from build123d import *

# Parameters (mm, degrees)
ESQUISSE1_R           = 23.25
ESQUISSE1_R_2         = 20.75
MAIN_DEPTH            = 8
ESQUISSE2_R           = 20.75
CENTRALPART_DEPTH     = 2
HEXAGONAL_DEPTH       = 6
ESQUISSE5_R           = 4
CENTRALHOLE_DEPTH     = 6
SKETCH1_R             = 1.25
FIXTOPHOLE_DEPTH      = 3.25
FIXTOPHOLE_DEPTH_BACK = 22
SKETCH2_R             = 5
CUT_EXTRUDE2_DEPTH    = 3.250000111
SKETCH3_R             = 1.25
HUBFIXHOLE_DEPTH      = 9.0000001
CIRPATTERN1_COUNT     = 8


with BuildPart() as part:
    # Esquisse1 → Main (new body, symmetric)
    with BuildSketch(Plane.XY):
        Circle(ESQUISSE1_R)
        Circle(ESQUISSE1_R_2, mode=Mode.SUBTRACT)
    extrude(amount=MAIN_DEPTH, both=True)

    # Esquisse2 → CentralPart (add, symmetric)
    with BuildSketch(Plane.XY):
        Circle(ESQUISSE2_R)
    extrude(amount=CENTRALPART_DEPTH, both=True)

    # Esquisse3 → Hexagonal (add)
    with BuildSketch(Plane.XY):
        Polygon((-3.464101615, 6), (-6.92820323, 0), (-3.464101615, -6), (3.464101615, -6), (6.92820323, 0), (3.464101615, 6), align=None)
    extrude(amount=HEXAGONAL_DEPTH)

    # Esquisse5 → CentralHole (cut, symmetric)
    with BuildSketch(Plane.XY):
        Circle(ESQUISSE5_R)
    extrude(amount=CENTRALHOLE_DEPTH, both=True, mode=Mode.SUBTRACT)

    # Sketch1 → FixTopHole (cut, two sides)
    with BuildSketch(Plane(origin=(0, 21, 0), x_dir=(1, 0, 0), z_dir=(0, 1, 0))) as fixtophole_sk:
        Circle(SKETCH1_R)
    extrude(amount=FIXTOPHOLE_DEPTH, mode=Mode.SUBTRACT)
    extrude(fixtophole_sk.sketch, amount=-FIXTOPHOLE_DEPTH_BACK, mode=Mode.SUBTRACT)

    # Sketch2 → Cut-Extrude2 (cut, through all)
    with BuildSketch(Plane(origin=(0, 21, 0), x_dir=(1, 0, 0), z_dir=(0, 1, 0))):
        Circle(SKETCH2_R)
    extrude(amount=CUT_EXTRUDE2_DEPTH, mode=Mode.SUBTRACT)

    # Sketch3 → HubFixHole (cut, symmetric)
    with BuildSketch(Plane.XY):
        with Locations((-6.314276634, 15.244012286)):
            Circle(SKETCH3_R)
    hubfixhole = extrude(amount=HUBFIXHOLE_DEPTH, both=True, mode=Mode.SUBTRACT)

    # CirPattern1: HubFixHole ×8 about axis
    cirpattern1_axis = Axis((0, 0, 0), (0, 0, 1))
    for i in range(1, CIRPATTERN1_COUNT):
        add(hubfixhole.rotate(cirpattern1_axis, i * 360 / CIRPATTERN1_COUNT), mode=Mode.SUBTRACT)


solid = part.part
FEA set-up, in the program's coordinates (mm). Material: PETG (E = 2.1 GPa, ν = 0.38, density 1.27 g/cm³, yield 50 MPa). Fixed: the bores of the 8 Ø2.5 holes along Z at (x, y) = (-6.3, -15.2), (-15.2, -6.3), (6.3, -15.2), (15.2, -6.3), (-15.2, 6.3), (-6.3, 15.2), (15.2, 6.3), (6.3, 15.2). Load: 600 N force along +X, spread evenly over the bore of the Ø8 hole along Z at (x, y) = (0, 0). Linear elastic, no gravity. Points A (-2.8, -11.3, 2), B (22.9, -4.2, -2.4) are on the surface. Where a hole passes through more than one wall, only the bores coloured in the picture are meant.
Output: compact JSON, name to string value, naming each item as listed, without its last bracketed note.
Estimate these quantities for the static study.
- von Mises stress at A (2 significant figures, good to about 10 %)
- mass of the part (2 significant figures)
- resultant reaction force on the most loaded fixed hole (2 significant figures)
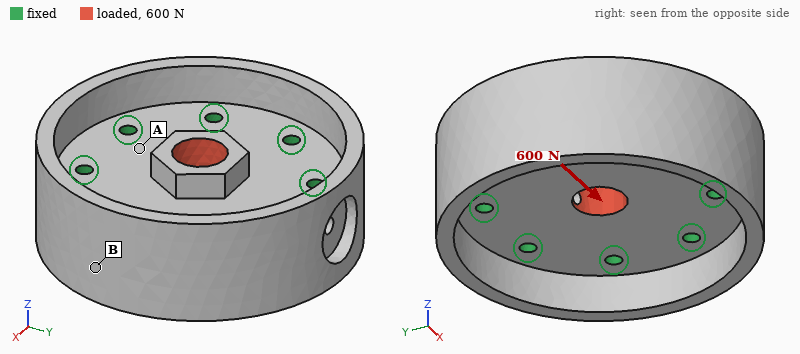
{"von Mises stress at A": "2.6 MPa", "mass of the part": "13 g", "resultant reaction force on the most loaded fixed hole": "120 N"}
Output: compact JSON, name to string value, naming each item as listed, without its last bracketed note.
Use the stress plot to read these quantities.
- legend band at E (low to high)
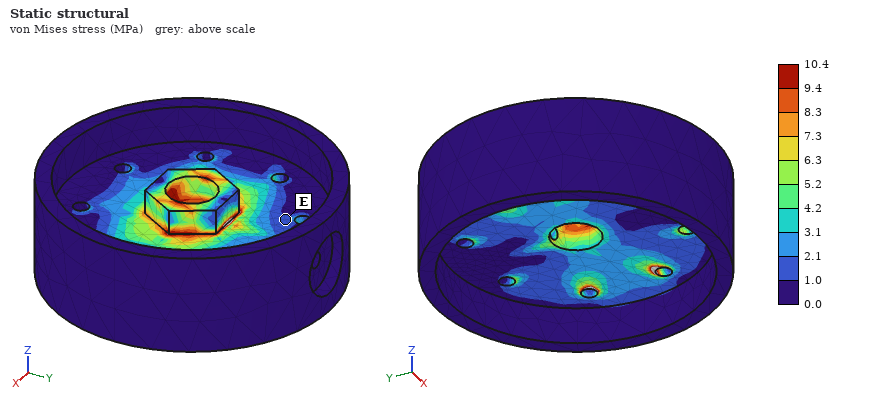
{"legend band at E": "1.0 to 2.1 MPa"}
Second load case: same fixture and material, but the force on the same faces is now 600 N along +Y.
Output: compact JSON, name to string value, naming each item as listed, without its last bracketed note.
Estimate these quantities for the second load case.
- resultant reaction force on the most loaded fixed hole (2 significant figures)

{"resultant reaction force on the most loaded fixed hole": "120 N"}
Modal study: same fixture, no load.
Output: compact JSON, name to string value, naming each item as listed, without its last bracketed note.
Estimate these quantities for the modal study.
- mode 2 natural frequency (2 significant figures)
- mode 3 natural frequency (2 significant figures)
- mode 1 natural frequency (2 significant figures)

{"mode 2 natural frequency": "5600 Hz", "mode 3 natural frequency": "6500 Hz", "mode 1 natural frequency": "5500 Hz"}
